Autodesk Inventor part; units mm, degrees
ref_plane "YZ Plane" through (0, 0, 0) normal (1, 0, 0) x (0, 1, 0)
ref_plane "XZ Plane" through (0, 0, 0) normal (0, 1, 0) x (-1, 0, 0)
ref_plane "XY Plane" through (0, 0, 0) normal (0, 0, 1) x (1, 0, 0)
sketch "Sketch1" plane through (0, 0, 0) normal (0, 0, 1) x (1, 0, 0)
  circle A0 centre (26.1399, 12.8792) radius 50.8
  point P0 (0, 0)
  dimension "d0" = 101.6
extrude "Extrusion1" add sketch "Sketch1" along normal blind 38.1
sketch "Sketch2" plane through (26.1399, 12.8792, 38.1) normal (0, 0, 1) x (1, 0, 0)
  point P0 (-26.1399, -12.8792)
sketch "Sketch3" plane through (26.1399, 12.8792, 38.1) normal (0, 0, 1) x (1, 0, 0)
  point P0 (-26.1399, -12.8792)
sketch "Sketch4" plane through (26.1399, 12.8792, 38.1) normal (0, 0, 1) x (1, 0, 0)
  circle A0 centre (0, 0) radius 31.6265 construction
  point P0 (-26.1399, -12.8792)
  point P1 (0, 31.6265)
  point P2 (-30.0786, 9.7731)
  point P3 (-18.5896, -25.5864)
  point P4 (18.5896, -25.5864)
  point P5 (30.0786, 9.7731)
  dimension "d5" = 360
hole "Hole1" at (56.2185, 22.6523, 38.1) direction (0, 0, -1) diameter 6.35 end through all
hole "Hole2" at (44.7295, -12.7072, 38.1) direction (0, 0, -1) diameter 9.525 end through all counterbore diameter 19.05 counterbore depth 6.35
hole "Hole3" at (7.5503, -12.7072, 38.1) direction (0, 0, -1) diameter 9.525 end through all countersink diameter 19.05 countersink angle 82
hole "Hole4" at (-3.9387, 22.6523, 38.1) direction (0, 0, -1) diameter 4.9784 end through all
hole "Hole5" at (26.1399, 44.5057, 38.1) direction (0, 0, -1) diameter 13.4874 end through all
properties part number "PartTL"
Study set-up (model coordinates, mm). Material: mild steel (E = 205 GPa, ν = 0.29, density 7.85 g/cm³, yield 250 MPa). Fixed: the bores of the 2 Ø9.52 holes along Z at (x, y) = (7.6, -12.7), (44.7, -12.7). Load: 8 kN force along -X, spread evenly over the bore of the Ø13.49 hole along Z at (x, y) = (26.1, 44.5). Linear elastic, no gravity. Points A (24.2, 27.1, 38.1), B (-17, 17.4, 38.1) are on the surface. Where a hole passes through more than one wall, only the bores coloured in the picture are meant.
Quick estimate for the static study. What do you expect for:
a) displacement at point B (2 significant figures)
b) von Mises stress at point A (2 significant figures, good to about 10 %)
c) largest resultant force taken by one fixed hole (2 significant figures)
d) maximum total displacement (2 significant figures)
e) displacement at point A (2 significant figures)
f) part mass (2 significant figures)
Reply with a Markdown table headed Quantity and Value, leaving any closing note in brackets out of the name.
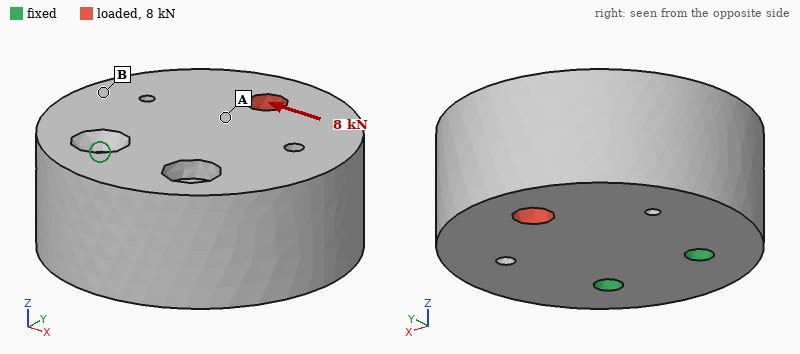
| Quantity | Value |
|---|---|
| displacement at point B | 3.7 µm |
| von Mises stress at point A | 7.6 MPa |
| largest resultant force taken by one fixed hole | 11 kN |
| maximum total displacement | 6.4 µm |
| displacement at point A | 3.4 µm |
| part mass | 2.3 kg |
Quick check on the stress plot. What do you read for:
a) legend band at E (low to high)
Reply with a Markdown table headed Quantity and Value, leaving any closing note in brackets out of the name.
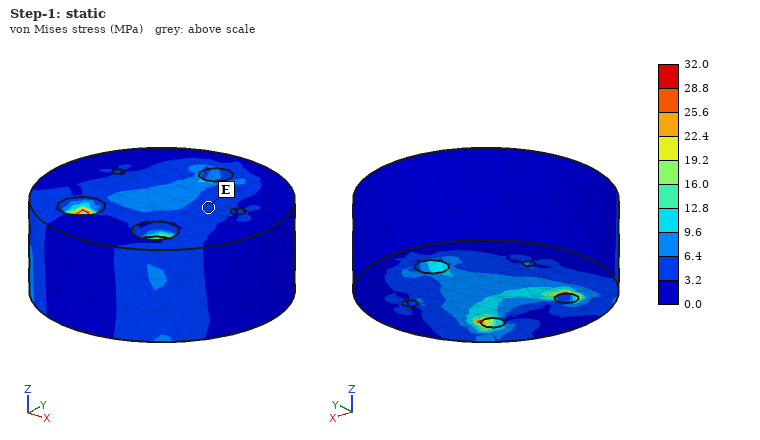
| Quantity | Value |
|---|---|
| legend band at E | 3.2 to 6.4 MPa |
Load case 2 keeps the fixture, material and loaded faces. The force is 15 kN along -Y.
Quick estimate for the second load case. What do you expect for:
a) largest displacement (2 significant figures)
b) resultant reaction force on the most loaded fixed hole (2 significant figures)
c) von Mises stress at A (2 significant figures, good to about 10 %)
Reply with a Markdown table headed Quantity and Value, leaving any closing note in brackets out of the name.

| Quantity | Value |
|---|---|
| largest displacement | 3.3 µm |
| resultant reaction force on the most loaded fixed hole | 7.6 kN |
| von Mises stress at A | 9.6 MPa |
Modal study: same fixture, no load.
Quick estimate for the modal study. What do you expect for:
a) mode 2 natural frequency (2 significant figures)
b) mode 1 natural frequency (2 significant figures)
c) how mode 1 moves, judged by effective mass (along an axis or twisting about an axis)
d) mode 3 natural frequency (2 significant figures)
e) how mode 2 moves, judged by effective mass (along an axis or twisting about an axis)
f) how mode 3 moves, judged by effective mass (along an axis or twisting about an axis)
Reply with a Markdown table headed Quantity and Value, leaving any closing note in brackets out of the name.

| Quantity | Value |
|---|---|
| mode 2 natural frequency | 6100 Hz |
| mode 1 natural frequency | 4400 Hz |
| how mode 1 moves, judged by effective mass | along Z |
| mode 3 natural frequency | 8100 Hz |
| how mode 2 moves, judged by effective mass | along X |
| how mode 3 moves, judged by effective mass | twisting about Y |
